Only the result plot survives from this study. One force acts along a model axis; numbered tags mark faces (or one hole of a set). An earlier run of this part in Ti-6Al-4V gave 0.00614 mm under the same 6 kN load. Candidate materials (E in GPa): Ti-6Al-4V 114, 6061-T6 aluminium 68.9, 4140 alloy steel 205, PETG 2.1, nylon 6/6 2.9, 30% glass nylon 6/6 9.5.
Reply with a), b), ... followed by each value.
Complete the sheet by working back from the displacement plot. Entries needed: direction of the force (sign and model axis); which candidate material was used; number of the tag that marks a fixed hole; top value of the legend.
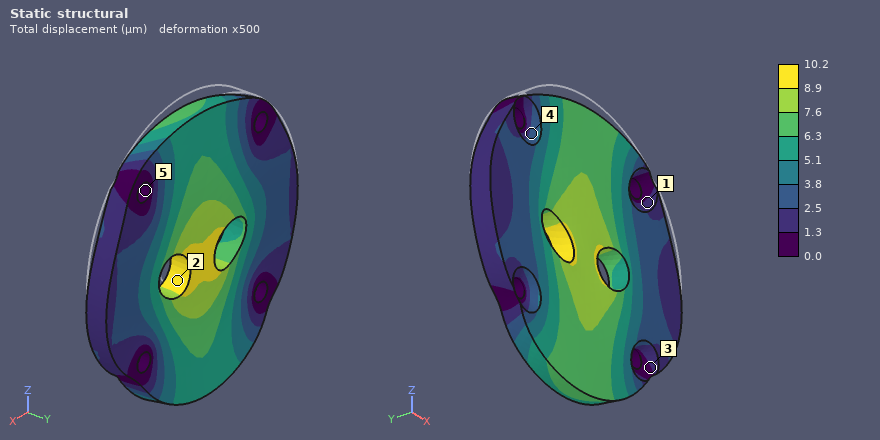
a) -Z
b) 6061-T6 aluminium
c) 5
d) 10.2 µm
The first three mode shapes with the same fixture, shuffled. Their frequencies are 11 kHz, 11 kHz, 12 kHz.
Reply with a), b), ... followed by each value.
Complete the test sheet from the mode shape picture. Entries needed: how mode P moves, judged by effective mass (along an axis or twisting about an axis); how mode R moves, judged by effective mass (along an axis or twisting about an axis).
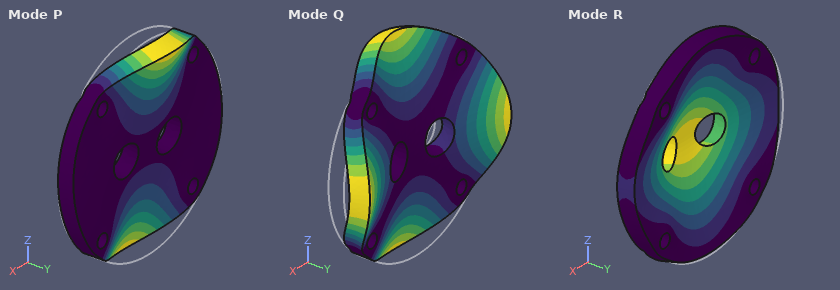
a) twisting about X
b) along Y
